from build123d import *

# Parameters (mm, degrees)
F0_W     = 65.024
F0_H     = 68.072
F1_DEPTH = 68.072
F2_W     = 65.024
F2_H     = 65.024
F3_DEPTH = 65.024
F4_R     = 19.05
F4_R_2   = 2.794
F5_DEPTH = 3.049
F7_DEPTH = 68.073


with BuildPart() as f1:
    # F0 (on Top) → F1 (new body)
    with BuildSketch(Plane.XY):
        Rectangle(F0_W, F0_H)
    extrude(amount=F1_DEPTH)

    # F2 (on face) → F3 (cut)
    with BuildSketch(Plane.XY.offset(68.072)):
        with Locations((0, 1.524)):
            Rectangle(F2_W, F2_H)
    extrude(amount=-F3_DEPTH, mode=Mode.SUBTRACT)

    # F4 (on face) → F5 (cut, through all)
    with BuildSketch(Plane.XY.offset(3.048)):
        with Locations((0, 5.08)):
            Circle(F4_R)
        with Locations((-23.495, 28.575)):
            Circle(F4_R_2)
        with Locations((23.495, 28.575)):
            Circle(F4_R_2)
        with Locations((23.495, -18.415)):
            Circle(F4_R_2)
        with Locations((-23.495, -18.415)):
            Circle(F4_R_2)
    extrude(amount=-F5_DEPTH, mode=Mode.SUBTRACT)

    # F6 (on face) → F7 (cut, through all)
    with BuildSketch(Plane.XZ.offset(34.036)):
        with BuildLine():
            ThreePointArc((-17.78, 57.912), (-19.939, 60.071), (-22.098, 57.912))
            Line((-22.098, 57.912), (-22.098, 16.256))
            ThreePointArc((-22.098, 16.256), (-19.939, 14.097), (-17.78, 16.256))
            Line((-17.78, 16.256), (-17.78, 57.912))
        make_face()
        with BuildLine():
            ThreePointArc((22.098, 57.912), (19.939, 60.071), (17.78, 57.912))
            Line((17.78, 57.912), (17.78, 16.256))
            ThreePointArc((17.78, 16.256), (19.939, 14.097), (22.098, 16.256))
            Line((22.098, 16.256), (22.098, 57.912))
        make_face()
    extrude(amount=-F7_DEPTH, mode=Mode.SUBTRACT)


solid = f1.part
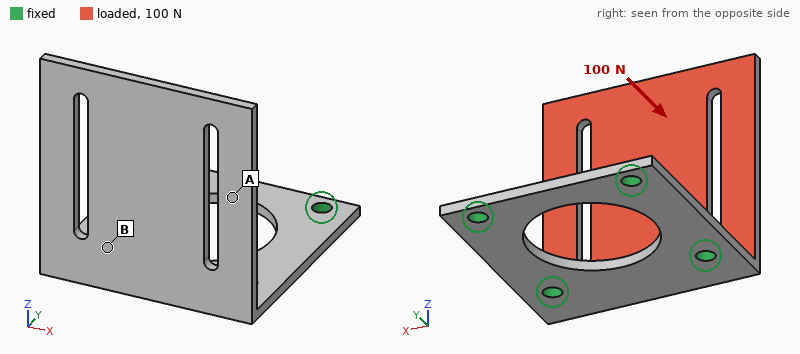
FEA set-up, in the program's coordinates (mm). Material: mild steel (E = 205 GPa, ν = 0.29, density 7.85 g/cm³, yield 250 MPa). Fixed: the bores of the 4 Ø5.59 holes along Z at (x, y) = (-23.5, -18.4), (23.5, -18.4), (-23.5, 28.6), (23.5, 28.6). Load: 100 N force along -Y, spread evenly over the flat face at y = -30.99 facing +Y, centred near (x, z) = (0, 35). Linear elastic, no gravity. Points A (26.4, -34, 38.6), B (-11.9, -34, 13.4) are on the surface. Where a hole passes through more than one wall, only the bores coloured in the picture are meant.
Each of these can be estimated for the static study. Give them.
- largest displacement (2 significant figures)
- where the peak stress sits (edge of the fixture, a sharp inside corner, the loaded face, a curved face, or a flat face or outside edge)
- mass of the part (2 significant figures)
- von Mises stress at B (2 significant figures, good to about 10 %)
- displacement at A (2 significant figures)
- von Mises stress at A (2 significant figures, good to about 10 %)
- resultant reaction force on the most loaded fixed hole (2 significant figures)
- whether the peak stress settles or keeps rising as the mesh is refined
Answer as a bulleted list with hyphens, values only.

- 0.22 mm
- edge of the fixture
- 170 g
- 22 MPa
- 0.10 mm
- 8.3 MPa
- 52 N
- keeps rising
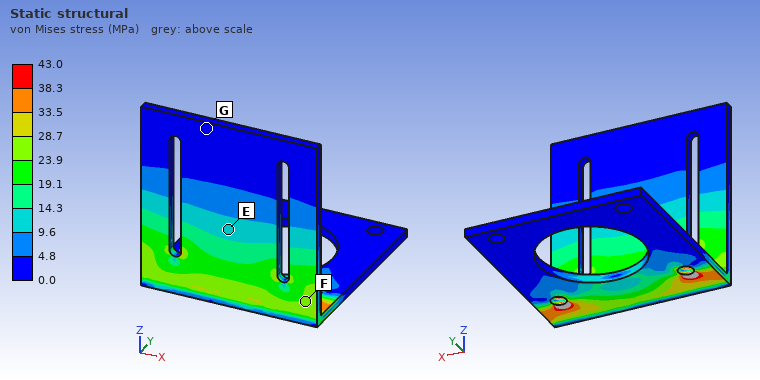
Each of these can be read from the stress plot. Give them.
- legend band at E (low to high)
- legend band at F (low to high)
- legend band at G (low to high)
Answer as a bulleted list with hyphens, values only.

- 9.6 to 14.3 MPa
- 23.9 to 28.7 MPa
- 0.0 to 4.8 MPa
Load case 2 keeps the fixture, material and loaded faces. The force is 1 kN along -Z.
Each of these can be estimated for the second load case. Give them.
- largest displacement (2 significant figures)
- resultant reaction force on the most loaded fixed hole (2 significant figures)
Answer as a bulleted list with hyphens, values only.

- 0.10 mm
- 510 N
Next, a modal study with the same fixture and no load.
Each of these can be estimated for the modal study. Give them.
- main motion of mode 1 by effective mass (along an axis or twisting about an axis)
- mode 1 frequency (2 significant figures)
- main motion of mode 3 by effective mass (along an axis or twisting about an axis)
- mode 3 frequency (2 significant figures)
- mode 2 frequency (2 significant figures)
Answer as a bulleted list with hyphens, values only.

- along Y
- 440 Hz
- along X
- 2000 Hz
- 1200 Hz
